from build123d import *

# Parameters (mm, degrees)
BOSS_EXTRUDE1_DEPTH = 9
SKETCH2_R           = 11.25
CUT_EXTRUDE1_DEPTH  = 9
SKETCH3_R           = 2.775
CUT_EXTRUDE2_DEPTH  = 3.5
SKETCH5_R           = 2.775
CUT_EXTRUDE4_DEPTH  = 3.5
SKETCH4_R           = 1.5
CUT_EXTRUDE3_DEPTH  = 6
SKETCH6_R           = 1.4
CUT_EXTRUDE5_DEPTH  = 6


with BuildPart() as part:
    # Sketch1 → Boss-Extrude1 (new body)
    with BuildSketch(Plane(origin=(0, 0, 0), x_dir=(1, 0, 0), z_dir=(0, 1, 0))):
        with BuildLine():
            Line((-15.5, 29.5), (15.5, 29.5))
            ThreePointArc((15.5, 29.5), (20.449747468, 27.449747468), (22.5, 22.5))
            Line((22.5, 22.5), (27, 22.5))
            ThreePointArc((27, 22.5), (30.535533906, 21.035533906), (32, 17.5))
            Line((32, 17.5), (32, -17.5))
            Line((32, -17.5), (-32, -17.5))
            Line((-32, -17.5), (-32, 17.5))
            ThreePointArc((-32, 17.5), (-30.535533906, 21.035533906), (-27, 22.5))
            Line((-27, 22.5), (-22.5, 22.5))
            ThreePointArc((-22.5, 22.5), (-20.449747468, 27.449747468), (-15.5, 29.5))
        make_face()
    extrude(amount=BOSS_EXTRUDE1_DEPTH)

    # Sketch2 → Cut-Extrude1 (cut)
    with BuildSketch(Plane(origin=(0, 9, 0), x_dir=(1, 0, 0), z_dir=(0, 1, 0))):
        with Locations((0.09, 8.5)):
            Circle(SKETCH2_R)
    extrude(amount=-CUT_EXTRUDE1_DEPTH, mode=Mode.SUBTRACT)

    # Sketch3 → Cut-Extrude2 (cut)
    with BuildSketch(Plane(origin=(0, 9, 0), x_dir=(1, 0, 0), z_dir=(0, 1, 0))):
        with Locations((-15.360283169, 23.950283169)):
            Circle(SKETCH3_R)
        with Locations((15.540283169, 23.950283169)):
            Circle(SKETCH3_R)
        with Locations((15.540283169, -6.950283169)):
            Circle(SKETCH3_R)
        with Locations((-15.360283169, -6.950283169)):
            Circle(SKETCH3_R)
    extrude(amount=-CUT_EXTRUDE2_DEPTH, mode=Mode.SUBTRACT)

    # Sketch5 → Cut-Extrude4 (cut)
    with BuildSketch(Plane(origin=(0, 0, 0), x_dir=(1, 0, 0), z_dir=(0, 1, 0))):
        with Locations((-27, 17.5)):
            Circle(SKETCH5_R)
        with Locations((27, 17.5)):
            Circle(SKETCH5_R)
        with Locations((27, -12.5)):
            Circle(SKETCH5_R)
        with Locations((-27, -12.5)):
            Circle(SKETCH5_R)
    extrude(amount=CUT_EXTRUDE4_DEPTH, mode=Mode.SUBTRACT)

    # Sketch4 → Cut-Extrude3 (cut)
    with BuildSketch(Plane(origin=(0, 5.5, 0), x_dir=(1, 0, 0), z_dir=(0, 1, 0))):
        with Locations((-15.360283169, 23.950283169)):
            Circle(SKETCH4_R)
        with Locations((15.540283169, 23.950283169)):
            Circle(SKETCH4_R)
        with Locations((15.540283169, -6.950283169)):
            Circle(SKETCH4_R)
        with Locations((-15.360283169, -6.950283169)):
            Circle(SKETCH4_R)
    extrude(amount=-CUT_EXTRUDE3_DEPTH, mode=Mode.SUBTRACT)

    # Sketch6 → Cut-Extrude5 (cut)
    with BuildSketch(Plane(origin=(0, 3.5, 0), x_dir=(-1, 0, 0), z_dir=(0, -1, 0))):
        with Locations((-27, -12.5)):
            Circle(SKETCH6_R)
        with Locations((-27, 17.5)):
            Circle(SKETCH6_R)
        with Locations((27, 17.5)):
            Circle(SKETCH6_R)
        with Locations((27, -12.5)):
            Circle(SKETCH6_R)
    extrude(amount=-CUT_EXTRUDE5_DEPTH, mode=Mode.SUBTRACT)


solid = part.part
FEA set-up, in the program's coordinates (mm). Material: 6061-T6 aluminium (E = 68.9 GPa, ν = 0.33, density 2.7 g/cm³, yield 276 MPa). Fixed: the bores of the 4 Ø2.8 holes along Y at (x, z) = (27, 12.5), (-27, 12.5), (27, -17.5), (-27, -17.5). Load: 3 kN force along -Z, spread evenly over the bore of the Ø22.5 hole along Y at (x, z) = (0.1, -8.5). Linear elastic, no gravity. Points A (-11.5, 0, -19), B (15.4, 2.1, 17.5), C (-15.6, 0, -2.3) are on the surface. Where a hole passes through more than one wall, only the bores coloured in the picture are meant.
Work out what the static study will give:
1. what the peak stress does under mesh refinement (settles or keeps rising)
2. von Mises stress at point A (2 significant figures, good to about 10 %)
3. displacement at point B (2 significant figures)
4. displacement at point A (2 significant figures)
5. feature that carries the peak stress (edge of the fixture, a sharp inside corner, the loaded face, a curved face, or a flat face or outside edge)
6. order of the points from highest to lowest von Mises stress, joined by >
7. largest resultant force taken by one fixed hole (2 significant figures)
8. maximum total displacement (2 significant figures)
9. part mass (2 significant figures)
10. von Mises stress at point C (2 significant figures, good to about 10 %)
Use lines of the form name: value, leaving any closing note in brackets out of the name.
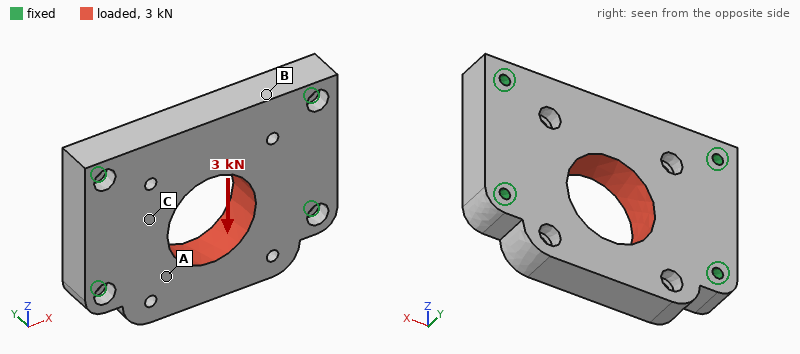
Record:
what the peak stress does under mesh refinement: keeps rising
von Mises stress at point A: 6.3 MPa
displacement at point B: 3.3 µm
displacement at point A: 4.8 µm
feature that carries the peak stress: edge of the fixture
order of the points from highest to lowest von Mises stress, joined by >: C > A > B
largest resultant force taken by one fixed hole: 840 N
maximum total displacement: 7.1 µm
part mass: 57 g
von Mises stress at point C: 9.9 MPa
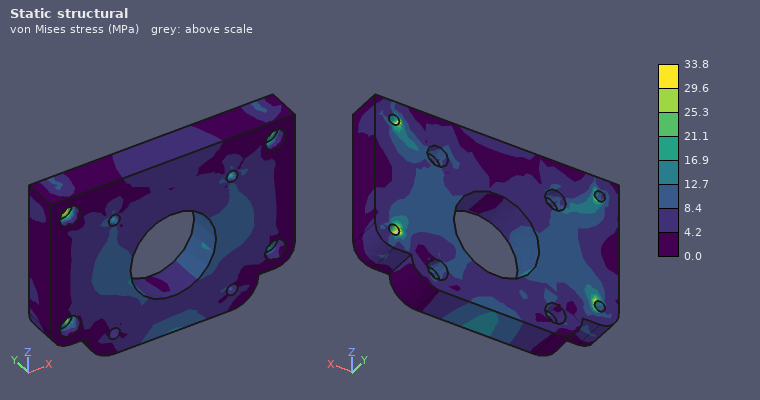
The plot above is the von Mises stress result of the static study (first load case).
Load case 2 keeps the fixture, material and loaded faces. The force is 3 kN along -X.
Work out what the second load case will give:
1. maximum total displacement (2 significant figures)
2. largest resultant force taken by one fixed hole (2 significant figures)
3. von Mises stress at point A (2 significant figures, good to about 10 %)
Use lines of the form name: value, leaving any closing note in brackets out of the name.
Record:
maximum total displacement: 3.5 µm
largest resultant force taken by one fixed hole: 920 N
von Mises stress at point A: 5.7 MPa
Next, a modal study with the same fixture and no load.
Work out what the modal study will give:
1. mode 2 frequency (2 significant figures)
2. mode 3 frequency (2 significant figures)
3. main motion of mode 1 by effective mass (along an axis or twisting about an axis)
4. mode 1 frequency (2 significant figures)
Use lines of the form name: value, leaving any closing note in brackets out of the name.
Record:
mode 2 frequency: 12 kHz
mode 3 frequency: 21 kHz
main motion of mode 1 by effective mass: along Y
mode 1 frequency: 9300 Hz
